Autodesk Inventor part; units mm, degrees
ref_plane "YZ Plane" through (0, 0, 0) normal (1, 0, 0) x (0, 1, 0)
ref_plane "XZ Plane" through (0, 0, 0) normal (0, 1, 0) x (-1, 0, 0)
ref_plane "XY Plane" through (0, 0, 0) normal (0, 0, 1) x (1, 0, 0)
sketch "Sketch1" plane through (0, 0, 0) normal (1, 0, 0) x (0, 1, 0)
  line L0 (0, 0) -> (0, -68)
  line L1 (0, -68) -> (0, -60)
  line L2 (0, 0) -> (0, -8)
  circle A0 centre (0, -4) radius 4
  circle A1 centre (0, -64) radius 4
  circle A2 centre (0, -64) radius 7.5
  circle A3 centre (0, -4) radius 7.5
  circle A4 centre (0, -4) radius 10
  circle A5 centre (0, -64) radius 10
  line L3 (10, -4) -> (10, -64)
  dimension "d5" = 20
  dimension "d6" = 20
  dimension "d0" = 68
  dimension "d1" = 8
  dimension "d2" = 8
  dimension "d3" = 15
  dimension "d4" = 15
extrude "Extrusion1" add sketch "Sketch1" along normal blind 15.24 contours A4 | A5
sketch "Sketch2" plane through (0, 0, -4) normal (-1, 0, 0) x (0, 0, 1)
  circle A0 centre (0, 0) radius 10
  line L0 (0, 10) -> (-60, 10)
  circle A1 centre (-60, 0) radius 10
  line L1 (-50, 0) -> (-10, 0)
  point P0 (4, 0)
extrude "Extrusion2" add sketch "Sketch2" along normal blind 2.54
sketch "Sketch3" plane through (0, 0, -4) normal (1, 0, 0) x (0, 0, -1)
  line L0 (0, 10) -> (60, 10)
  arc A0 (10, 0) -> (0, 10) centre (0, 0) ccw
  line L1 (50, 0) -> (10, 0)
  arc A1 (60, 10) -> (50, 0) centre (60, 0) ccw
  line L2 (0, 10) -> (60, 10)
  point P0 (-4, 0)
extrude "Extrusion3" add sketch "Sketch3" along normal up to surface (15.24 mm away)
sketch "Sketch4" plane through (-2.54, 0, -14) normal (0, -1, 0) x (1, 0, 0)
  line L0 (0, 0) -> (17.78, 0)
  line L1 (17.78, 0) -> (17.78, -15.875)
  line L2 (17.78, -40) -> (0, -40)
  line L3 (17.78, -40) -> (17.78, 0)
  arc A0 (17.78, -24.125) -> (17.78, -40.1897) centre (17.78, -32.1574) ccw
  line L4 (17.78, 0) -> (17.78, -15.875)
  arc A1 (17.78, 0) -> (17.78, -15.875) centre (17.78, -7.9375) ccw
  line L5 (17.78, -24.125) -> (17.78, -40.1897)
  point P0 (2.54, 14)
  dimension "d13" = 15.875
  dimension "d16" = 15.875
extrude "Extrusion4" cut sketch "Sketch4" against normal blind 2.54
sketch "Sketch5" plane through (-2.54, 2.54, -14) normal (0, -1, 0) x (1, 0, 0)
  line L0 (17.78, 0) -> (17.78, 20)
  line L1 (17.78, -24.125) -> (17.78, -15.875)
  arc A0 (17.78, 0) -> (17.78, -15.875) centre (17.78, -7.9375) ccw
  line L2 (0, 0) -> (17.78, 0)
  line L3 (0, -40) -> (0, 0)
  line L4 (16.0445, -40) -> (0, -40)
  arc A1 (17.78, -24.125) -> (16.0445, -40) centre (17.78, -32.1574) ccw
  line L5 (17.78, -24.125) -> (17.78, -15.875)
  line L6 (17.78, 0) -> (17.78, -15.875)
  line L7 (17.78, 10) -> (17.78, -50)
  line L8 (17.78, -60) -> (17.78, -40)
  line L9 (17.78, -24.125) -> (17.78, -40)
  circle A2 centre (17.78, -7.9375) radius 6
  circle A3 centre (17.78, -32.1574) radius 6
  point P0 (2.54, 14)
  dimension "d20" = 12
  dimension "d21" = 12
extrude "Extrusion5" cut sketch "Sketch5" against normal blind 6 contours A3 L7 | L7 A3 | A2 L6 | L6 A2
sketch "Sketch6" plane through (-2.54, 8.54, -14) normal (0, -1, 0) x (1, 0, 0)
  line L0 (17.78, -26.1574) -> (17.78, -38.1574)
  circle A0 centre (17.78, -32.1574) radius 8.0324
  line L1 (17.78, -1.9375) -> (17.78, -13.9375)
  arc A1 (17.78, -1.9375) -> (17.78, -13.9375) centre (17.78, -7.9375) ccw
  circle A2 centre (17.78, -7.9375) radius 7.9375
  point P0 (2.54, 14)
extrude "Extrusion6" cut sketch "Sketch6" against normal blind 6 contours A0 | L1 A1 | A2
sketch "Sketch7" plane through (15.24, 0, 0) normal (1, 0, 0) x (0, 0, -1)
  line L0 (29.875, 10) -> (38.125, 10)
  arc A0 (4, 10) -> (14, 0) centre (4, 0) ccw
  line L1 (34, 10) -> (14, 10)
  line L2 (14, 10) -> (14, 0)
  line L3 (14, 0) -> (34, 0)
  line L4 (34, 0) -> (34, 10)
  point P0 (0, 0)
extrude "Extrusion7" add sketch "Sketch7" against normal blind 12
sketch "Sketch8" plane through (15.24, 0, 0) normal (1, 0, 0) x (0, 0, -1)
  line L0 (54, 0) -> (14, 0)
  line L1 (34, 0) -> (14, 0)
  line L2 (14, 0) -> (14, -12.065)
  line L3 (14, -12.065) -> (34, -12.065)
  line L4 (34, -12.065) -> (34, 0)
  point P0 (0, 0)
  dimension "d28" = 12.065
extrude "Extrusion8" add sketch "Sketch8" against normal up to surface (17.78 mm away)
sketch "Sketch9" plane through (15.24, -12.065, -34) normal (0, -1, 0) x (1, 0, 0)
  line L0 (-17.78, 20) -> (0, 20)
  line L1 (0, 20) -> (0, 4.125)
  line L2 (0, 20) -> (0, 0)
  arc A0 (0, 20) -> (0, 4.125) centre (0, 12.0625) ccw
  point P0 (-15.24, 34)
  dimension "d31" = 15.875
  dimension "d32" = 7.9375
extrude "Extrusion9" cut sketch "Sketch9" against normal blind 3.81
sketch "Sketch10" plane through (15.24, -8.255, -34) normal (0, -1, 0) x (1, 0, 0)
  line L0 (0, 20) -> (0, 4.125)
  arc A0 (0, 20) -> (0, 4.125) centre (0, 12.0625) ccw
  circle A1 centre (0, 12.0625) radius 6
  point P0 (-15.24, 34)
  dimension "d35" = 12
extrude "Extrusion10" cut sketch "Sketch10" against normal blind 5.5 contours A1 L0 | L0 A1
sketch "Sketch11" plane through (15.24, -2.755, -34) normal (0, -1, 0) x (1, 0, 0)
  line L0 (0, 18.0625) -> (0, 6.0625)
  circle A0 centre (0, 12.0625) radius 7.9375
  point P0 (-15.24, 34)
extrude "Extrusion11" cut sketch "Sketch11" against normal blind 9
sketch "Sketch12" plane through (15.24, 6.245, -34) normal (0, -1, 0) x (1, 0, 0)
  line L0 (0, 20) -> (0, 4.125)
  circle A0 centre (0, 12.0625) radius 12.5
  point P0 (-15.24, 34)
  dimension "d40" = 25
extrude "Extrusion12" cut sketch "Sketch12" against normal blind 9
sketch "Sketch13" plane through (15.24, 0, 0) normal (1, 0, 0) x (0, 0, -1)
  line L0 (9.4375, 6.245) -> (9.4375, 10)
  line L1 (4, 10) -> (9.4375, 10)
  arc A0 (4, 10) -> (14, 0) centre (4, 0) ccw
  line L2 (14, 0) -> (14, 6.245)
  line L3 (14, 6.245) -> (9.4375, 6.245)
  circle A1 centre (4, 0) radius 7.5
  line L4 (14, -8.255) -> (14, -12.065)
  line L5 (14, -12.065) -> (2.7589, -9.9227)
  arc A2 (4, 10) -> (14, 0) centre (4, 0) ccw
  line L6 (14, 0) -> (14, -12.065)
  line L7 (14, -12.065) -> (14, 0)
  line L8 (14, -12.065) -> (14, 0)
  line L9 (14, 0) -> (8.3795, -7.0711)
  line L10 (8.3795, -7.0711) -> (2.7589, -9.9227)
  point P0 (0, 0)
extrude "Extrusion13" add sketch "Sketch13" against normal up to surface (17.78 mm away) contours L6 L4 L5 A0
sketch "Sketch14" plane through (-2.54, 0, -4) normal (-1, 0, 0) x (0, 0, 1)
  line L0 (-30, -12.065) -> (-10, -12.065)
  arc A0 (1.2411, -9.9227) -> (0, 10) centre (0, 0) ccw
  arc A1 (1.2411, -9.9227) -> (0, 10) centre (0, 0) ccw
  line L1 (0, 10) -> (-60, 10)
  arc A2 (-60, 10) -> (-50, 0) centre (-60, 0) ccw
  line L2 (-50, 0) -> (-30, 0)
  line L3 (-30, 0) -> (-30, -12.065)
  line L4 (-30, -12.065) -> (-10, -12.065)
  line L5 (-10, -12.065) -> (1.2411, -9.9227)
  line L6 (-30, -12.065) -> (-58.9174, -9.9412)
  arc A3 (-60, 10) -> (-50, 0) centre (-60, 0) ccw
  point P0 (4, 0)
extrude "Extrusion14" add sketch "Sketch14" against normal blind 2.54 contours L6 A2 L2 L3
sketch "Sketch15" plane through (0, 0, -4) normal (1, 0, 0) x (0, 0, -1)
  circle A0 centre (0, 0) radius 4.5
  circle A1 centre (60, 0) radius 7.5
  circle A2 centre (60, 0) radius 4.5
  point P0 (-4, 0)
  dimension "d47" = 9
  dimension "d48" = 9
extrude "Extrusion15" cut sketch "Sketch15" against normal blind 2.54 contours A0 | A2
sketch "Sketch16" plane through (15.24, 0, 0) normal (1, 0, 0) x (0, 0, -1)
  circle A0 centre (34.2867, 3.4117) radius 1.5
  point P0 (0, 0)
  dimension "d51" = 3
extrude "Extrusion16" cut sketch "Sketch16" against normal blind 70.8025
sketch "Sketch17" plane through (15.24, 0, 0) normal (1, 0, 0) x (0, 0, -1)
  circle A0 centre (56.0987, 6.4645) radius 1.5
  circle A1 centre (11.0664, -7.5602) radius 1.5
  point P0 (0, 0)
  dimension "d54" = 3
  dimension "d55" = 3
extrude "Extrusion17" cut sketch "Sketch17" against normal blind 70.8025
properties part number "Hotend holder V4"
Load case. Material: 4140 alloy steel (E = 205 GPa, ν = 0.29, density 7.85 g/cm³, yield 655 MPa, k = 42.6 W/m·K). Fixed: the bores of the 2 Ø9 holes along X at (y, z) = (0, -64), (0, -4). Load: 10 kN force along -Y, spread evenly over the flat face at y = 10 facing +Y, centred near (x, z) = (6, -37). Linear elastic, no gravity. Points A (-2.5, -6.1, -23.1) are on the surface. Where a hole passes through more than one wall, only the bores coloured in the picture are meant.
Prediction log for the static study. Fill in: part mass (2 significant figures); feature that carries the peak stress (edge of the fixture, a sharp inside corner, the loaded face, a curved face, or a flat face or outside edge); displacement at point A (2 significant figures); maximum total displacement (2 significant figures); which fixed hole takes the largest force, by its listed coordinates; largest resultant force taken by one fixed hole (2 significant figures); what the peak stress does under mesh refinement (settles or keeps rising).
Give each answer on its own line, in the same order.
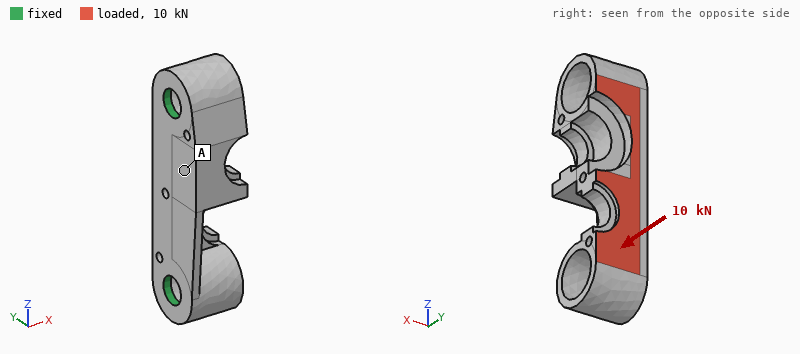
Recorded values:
120 g
edge of the fixture
17 µm
74 µm
(0, -64)
5.6 kN
keeps rising
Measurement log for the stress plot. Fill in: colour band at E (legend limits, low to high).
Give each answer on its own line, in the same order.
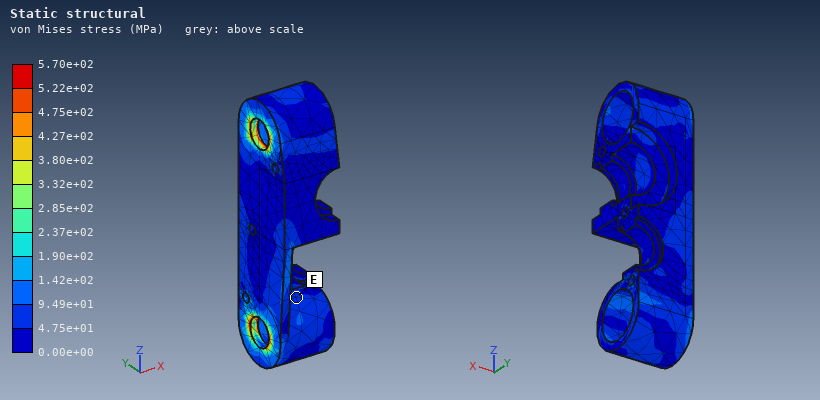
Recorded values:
4.75e+01 to 9.49e+01 MPa
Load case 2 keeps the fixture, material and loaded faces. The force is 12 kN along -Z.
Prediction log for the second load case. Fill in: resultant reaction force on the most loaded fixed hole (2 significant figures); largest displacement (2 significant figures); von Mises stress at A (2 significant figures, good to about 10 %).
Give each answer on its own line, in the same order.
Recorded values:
6.6 kN
18 µm
31 MPa
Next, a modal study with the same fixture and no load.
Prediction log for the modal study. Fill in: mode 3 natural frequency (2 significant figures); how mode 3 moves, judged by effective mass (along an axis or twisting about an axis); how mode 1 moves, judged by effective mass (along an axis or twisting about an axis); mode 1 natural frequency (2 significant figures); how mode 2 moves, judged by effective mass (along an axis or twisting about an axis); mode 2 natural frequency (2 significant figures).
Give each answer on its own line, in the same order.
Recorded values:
14 kHz
along Y
along Y
7100 Hz
along X
8100 Hz
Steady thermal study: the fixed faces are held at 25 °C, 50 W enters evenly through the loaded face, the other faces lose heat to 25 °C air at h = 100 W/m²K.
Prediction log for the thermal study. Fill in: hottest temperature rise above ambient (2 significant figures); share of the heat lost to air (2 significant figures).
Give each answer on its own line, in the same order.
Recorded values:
56 K
40 %
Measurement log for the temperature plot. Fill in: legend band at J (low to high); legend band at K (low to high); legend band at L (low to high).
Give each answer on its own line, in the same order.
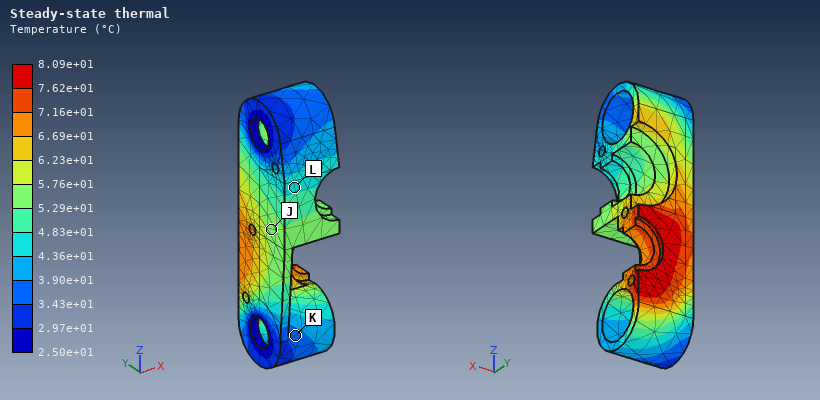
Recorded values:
5.29e+01 to 5.76e+01 °C
3.43e+01 to 3.90e+01 °C
4.36e+01 to 4.83e+01 °C
